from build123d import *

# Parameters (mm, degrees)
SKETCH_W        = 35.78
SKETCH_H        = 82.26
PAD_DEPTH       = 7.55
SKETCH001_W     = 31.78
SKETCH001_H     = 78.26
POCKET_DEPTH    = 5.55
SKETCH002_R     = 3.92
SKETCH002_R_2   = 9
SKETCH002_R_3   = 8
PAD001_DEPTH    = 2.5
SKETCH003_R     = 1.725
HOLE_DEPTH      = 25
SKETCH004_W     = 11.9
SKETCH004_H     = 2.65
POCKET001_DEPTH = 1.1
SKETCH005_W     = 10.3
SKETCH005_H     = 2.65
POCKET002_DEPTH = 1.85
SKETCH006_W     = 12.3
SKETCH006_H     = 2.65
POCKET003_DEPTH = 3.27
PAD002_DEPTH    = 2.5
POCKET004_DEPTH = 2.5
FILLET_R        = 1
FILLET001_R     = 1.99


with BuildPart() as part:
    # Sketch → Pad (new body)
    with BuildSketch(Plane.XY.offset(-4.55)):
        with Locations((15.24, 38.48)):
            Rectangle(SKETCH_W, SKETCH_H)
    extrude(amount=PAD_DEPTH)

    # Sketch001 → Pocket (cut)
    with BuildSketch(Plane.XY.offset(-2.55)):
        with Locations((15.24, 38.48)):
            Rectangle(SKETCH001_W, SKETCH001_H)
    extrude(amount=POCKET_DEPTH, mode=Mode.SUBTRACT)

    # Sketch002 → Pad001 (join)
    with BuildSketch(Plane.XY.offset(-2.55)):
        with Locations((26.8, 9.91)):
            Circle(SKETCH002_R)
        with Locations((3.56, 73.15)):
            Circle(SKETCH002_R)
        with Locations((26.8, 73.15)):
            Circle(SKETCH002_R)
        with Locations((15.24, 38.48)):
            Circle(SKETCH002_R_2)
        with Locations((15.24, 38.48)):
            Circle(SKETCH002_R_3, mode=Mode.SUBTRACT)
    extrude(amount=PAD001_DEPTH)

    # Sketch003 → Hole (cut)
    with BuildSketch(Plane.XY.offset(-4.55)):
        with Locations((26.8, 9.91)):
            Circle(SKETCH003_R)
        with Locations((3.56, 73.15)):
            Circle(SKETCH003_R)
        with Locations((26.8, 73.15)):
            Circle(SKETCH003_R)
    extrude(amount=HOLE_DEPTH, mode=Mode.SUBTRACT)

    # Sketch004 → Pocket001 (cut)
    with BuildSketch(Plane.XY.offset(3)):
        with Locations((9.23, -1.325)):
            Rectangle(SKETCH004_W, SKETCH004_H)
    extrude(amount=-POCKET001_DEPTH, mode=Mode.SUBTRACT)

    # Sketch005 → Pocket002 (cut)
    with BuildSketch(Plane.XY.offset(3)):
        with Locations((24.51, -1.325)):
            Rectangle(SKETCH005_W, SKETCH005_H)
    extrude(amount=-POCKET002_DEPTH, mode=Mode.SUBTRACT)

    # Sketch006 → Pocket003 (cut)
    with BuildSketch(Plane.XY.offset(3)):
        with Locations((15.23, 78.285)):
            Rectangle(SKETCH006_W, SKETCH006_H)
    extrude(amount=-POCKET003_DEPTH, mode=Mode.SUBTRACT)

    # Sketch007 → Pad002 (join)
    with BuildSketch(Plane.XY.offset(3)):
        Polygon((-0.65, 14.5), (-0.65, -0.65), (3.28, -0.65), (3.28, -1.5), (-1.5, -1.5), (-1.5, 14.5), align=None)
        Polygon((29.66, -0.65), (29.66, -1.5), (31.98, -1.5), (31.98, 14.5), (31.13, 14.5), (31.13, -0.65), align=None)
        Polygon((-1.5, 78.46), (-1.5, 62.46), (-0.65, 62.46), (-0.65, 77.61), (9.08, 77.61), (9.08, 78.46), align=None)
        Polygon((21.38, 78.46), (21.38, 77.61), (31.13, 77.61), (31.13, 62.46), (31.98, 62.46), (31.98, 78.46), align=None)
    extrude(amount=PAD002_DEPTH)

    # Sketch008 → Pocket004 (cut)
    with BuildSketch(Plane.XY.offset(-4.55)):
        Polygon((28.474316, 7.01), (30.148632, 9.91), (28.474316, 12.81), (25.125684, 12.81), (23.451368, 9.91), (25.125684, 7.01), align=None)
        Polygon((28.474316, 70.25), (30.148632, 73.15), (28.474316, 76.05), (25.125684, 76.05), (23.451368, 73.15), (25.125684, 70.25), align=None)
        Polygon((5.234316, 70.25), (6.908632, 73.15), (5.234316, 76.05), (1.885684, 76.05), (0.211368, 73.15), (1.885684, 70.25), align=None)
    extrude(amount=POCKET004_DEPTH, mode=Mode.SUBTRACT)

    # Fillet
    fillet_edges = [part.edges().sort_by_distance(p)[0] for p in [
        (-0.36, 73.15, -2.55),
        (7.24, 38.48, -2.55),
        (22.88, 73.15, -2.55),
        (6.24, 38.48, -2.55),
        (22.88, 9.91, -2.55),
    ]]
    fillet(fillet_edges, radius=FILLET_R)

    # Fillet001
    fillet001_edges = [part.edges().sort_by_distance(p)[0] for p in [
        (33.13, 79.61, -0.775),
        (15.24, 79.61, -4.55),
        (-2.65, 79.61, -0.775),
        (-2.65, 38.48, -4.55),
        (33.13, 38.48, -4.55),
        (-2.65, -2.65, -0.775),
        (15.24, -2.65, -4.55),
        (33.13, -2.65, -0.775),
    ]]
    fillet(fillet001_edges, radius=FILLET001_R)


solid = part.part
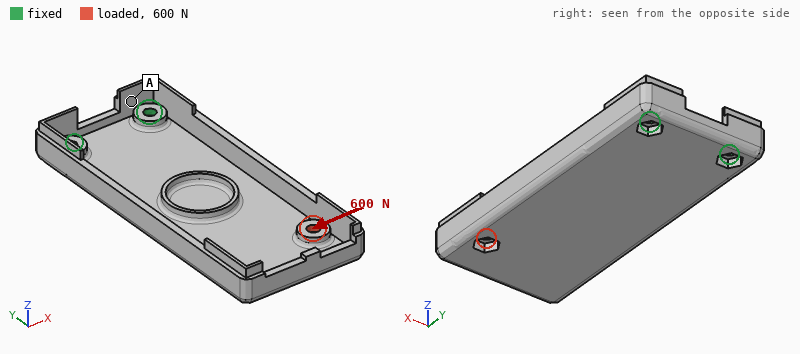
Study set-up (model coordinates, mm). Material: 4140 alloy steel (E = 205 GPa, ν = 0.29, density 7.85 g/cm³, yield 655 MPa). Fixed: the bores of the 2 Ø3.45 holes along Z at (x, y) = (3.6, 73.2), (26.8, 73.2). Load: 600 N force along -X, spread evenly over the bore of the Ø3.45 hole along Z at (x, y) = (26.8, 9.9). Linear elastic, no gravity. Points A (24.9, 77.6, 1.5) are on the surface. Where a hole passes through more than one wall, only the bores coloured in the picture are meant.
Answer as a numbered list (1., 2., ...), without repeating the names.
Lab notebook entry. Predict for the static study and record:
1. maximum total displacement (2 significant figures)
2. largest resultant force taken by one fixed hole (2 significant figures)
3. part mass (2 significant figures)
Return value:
1. 0.22 mm
2. 1.5 kN
3. 67 g
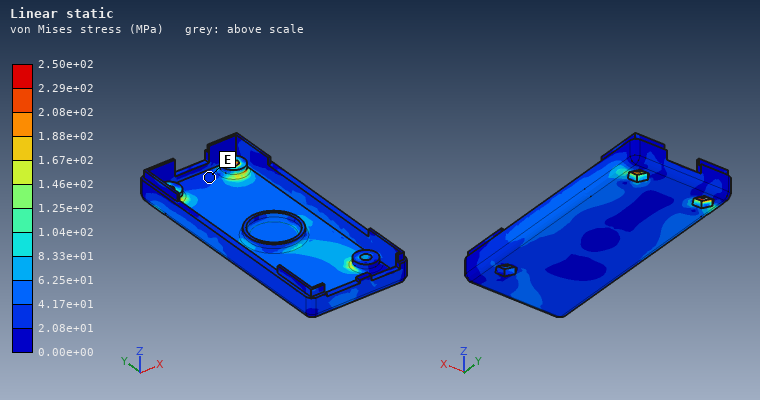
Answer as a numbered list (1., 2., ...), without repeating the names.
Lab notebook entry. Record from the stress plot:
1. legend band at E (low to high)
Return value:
1. 2.08e+01 to 4.17e+01 MPa
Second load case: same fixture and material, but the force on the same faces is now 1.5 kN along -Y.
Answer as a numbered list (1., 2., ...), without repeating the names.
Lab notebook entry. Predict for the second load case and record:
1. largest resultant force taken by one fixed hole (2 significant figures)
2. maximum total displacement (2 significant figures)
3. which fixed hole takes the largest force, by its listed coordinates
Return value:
1. 1.4 kN
2. 0.16 mm
3. (26.8, 73.2)
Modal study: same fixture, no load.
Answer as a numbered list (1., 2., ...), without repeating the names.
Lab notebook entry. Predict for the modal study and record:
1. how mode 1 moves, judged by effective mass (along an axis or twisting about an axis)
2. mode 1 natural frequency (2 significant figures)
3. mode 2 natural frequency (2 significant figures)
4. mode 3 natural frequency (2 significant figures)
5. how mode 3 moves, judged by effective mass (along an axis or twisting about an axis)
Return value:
1. along Z
2. 580 Hz
3. 1300 Hz
4. 3400 Hz
5. along X
